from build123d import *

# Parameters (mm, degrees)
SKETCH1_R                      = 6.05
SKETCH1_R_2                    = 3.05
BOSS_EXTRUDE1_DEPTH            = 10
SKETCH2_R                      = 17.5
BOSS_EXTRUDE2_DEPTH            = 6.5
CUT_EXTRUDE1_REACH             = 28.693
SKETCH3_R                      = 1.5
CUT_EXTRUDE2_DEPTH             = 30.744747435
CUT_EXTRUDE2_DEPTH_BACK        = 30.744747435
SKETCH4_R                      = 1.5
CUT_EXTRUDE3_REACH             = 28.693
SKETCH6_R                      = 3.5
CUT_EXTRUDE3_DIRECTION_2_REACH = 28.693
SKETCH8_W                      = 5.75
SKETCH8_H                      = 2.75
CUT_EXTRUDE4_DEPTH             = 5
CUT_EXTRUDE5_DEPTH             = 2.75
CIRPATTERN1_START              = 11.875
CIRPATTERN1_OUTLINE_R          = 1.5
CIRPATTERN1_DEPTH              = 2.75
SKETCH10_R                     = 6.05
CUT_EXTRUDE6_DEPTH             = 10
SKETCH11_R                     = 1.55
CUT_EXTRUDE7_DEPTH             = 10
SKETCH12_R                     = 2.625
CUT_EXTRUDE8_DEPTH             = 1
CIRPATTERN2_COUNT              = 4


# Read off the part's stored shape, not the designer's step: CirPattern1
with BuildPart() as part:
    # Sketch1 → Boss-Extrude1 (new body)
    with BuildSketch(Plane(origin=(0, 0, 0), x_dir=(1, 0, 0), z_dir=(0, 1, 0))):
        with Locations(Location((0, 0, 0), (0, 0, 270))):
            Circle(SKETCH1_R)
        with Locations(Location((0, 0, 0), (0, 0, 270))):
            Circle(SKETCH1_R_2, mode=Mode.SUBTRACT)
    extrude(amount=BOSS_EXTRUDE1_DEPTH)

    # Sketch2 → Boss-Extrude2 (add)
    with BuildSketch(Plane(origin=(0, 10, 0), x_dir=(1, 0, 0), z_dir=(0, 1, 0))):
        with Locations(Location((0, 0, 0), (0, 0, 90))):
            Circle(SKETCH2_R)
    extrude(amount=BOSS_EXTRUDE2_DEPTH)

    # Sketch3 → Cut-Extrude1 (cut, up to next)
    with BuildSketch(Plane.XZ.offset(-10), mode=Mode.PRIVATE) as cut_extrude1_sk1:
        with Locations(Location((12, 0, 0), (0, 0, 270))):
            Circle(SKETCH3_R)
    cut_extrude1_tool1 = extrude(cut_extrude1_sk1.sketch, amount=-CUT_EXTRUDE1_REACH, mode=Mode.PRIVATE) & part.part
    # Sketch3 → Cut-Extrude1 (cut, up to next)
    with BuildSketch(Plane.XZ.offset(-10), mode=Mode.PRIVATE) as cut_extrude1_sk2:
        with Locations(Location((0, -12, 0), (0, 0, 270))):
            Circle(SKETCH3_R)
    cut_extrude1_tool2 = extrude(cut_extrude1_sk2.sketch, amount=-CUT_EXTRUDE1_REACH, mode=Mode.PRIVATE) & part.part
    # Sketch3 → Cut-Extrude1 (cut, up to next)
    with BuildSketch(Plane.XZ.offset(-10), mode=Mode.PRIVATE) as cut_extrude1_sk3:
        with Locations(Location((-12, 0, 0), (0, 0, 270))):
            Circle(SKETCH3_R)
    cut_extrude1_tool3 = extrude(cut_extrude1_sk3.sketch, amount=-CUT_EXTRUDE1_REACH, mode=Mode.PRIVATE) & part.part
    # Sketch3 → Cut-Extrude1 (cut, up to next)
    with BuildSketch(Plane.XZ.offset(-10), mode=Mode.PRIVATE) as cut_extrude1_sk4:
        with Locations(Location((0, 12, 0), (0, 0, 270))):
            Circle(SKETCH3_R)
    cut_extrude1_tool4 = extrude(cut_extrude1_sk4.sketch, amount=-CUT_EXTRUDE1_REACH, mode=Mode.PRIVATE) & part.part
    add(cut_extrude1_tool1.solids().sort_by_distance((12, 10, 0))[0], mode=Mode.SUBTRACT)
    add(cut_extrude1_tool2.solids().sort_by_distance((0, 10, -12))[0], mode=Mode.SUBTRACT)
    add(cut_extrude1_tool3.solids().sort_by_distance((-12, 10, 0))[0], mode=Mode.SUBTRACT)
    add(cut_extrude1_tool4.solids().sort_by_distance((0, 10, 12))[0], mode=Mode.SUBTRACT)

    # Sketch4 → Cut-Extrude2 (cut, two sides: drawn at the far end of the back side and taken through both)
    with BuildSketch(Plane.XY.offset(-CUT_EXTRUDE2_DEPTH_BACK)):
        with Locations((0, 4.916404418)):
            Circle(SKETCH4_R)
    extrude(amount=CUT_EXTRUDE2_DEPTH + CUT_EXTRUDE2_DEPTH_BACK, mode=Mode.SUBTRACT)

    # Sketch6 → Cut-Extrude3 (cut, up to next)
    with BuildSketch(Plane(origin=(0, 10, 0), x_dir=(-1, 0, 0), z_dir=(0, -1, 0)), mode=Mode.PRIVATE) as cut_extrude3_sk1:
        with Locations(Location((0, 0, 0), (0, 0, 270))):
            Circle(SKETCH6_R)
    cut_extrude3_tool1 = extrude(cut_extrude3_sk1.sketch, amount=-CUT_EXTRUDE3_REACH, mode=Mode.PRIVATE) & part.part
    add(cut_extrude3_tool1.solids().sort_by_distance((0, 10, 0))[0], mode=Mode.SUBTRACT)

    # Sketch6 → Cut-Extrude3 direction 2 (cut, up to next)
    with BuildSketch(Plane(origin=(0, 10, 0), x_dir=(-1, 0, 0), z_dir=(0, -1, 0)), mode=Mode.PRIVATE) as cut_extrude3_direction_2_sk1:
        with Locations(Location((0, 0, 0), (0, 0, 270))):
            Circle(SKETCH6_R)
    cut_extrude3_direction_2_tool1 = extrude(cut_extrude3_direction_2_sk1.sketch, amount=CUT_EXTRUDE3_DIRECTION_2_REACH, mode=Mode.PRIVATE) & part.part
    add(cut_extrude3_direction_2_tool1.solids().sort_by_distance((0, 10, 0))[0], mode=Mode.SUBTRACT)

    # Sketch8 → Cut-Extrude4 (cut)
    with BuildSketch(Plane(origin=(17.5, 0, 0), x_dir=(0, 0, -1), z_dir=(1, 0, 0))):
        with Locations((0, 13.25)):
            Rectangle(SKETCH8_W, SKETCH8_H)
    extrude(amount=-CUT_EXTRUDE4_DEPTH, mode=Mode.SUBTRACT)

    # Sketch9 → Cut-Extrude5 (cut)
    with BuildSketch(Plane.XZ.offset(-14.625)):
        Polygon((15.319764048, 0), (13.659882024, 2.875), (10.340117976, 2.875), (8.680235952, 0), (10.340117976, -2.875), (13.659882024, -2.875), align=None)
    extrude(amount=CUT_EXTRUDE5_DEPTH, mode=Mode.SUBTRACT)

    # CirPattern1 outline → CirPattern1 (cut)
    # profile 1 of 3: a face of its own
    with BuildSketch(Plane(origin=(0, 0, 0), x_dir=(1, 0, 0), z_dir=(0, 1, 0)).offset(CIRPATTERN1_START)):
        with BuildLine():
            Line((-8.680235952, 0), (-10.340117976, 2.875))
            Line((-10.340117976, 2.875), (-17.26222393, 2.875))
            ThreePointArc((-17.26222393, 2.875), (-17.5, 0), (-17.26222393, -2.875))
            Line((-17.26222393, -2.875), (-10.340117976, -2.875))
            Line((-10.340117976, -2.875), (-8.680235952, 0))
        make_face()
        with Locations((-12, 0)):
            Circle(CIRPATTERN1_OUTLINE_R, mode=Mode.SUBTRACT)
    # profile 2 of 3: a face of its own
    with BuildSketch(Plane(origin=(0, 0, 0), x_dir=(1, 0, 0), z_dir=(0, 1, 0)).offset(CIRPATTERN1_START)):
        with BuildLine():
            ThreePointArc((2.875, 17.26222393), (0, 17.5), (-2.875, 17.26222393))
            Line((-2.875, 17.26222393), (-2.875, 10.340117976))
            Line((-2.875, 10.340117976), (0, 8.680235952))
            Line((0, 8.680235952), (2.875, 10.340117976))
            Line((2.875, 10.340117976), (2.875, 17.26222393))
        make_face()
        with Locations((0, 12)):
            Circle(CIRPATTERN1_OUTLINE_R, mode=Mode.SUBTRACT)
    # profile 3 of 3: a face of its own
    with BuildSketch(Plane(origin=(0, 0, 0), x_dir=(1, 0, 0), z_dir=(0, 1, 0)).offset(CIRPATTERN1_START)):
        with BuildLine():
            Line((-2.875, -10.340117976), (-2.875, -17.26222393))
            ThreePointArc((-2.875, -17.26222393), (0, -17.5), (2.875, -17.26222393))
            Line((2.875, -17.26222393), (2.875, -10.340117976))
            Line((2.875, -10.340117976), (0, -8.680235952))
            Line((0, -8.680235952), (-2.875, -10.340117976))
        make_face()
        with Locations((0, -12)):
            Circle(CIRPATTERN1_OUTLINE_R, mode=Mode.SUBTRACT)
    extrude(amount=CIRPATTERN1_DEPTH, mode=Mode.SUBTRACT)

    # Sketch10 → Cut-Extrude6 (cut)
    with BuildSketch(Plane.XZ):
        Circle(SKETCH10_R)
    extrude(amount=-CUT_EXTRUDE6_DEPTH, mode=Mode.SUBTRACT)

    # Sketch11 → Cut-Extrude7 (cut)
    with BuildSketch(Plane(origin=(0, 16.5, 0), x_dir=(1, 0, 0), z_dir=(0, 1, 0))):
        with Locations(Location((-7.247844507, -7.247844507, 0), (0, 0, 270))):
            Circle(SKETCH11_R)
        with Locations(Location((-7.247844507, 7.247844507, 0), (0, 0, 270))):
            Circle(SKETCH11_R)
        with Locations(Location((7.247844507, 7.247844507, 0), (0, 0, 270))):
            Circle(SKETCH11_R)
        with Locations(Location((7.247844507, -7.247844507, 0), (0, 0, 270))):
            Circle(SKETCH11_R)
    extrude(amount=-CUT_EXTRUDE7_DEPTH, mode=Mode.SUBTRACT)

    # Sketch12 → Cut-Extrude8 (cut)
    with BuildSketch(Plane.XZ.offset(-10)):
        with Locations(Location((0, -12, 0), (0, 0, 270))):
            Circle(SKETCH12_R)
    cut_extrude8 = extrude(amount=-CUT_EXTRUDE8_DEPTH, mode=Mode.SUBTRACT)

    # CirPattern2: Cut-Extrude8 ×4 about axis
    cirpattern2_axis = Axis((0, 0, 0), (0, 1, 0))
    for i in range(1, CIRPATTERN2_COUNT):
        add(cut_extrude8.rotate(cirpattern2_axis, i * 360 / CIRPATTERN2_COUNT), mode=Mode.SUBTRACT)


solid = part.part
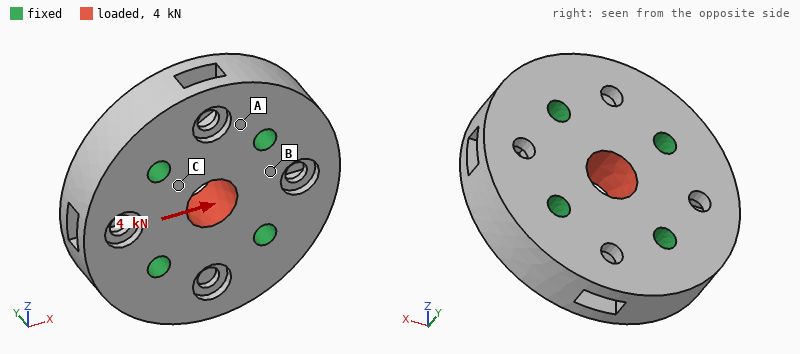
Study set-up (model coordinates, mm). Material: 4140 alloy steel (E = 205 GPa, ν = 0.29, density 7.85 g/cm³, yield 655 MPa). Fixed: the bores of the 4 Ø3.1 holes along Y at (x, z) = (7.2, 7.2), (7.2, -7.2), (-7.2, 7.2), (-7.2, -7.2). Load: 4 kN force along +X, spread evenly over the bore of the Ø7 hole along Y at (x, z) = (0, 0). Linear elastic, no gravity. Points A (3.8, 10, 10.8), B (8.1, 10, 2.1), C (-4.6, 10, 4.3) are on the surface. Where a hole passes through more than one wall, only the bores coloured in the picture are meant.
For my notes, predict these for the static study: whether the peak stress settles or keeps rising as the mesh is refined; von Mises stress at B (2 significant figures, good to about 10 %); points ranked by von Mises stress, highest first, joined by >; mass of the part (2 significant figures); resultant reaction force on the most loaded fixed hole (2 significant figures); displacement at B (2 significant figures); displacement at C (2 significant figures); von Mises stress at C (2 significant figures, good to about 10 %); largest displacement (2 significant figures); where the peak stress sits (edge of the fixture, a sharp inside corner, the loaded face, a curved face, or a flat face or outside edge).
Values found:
keeps rising
19 MPa
C > B > A
40 g
1.1 kN
0.63 µm
0.46 µm
27 MPa
1.2 µm
edge of the fixture
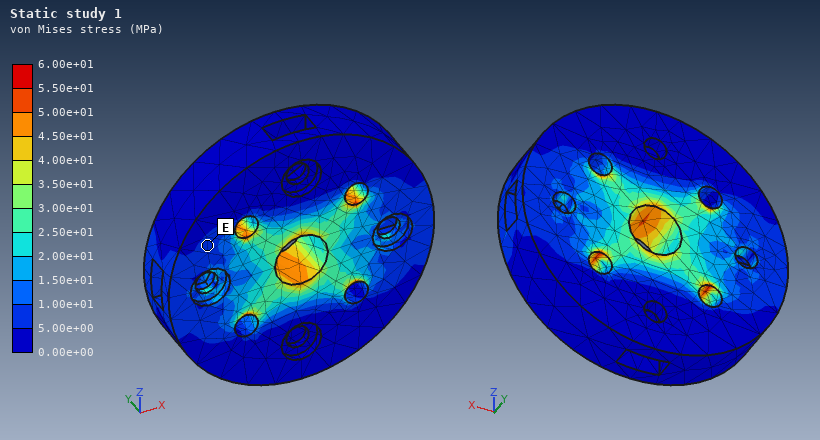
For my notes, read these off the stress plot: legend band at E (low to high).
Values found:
5.00e+00 to 1.00e+01 MPa
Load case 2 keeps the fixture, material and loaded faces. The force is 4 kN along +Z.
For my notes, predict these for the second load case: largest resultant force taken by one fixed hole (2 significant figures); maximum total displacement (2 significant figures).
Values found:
1.1 kN
1.2 µm
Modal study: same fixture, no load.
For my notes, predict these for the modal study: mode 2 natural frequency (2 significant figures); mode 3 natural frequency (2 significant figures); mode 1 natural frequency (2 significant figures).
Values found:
49 kHz
49 kHz
47 kHz
